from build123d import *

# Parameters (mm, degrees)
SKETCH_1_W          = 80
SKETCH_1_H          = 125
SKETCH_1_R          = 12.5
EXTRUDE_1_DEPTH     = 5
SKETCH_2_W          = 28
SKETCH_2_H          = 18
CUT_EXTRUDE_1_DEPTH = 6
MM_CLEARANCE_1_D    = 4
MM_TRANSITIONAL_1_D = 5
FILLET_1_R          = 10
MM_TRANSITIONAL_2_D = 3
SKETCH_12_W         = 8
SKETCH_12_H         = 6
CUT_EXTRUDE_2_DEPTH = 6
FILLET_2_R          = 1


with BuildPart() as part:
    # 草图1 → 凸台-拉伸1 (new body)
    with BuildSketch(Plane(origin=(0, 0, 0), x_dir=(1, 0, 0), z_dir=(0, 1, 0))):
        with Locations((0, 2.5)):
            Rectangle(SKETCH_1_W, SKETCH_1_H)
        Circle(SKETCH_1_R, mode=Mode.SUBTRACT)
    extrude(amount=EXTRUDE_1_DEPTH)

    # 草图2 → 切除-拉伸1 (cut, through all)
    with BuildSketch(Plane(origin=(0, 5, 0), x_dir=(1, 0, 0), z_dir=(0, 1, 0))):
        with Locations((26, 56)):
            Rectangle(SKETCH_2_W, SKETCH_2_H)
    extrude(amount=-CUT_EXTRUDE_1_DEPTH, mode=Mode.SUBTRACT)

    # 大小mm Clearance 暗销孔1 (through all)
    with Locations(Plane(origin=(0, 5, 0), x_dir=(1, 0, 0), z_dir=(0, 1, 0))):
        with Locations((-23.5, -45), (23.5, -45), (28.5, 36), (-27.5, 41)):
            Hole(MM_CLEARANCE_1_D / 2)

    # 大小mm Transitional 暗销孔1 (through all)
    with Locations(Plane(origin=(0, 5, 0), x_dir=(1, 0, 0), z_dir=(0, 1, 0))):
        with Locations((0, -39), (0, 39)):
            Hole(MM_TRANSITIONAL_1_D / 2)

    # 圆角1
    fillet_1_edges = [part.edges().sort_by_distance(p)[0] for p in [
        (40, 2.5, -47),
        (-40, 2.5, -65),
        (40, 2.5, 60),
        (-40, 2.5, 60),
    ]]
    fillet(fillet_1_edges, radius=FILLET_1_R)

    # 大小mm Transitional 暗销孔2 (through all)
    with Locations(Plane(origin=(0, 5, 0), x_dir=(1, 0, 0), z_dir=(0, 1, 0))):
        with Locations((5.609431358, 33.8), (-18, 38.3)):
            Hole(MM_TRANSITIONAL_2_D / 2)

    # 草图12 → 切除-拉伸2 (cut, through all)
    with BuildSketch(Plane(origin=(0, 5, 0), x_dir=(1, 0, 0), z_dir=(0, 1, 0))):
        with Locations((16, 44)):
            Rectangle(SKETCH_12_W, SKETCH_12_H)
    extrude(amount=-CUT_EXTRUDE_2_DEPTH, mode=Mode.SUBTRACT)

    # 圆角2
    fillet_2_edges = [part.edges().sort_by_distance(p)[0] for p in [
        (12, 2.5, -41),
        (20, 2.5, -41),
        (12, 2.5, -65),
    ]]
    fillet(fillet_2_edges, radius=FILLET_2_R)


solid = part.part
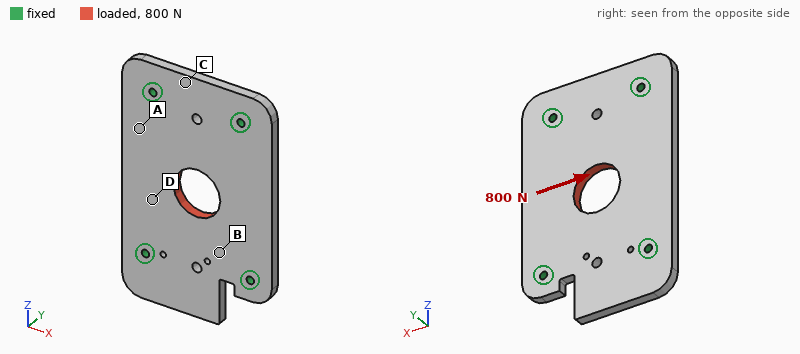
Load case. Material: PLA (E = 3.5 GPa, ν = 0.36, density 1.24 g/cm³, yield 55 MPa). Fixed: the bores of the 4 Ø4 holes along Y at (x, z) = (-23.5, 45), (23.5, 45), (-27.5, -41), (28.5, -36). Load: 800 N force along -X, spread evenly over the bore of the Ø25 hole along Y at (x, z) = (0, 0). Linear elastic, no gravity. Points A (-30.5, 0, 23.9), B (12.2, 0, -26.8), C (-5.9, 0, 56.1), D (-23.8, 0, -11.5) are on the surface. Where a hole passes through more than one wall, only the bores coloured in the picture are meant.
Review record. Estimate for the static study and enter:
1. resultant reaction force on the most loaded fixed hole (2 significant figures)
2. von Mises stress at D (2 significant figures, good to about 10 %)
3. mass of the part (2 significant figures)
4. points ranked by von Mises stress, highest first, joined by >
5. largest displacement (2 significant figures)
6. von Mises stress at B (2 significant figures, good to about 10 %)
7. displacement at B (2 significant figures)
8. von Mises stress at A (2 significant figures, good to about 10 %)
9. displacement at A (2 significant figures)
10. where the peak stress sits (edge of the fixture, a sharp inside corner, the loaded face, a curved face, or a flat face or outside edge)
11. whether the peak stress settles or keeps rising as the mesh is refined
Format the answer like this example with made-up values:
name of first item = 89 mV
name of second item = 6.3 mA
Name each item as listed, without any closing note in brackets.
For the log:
resultant reaction force on the most loaded fixed hole = 250 N
von Mises stress at D = 1.7 MPa
mass of the part = 54 g
points ranked by von Mises stress, highest first, joined by > = B > D > A > C
largest displacement = 46 µm
von Mises stress at B = 2.5 MPa
displacement at B = 18 µm
von Mises stress at A = 1.1 MPa
displacement at A = 27 µm
where the peak stress sits = edge of the fixture
whether the peak stress settles or keeps rising as the mesh is refined = keeps rising
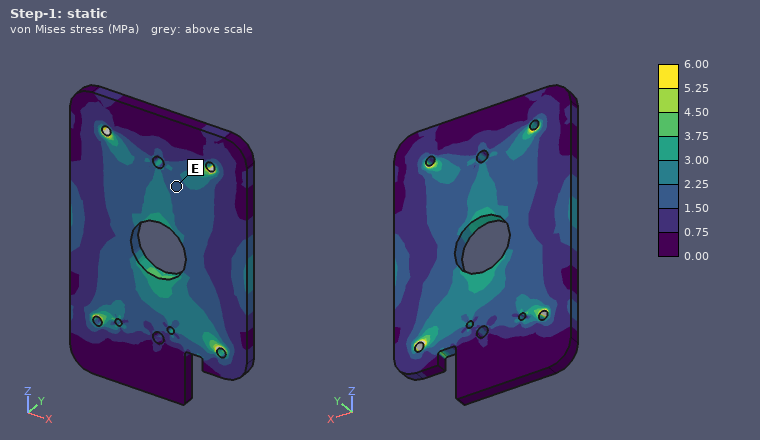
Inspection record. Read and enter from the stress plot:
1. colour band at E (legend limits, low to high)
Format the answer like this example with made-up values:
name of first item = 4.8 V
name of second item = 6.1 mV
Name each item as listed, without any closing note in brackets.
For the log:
colour band at E = 1.50 to 2.25 MPa
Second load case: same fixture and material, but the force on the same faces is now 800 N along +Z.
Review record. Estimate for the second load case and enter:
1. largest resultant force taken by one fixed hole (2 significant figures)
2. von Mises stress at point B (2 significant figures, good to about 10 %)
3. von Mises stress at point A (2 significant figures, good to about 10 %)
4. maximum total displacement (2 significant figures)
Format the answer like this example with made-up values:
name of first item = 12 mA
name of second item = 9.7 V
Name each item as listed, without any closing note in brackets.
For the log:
largest resultant force taken by one fixed hole = 220 N
von Mises stress at point B = 1.5 MPa
von Mises stress at point A = 0.73 MPa
maximum total displacement = 27 µm
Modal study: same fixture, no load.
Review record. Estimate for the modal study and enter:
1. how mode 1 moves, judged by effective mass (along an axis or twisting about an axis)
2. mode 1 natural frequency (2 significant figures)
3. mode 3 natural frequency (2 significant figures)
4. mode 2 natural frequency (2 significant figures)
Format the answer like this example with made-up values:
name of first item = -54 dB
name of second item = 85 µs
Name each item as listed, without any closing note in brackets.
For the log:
how mode 1 moves, judged by effective mass = along Y
mode 1 natural frequency = 1000 Hz
mode 3 natural frequency = 1400 Hz
mode 2 natural frequency = 1300 Hz
